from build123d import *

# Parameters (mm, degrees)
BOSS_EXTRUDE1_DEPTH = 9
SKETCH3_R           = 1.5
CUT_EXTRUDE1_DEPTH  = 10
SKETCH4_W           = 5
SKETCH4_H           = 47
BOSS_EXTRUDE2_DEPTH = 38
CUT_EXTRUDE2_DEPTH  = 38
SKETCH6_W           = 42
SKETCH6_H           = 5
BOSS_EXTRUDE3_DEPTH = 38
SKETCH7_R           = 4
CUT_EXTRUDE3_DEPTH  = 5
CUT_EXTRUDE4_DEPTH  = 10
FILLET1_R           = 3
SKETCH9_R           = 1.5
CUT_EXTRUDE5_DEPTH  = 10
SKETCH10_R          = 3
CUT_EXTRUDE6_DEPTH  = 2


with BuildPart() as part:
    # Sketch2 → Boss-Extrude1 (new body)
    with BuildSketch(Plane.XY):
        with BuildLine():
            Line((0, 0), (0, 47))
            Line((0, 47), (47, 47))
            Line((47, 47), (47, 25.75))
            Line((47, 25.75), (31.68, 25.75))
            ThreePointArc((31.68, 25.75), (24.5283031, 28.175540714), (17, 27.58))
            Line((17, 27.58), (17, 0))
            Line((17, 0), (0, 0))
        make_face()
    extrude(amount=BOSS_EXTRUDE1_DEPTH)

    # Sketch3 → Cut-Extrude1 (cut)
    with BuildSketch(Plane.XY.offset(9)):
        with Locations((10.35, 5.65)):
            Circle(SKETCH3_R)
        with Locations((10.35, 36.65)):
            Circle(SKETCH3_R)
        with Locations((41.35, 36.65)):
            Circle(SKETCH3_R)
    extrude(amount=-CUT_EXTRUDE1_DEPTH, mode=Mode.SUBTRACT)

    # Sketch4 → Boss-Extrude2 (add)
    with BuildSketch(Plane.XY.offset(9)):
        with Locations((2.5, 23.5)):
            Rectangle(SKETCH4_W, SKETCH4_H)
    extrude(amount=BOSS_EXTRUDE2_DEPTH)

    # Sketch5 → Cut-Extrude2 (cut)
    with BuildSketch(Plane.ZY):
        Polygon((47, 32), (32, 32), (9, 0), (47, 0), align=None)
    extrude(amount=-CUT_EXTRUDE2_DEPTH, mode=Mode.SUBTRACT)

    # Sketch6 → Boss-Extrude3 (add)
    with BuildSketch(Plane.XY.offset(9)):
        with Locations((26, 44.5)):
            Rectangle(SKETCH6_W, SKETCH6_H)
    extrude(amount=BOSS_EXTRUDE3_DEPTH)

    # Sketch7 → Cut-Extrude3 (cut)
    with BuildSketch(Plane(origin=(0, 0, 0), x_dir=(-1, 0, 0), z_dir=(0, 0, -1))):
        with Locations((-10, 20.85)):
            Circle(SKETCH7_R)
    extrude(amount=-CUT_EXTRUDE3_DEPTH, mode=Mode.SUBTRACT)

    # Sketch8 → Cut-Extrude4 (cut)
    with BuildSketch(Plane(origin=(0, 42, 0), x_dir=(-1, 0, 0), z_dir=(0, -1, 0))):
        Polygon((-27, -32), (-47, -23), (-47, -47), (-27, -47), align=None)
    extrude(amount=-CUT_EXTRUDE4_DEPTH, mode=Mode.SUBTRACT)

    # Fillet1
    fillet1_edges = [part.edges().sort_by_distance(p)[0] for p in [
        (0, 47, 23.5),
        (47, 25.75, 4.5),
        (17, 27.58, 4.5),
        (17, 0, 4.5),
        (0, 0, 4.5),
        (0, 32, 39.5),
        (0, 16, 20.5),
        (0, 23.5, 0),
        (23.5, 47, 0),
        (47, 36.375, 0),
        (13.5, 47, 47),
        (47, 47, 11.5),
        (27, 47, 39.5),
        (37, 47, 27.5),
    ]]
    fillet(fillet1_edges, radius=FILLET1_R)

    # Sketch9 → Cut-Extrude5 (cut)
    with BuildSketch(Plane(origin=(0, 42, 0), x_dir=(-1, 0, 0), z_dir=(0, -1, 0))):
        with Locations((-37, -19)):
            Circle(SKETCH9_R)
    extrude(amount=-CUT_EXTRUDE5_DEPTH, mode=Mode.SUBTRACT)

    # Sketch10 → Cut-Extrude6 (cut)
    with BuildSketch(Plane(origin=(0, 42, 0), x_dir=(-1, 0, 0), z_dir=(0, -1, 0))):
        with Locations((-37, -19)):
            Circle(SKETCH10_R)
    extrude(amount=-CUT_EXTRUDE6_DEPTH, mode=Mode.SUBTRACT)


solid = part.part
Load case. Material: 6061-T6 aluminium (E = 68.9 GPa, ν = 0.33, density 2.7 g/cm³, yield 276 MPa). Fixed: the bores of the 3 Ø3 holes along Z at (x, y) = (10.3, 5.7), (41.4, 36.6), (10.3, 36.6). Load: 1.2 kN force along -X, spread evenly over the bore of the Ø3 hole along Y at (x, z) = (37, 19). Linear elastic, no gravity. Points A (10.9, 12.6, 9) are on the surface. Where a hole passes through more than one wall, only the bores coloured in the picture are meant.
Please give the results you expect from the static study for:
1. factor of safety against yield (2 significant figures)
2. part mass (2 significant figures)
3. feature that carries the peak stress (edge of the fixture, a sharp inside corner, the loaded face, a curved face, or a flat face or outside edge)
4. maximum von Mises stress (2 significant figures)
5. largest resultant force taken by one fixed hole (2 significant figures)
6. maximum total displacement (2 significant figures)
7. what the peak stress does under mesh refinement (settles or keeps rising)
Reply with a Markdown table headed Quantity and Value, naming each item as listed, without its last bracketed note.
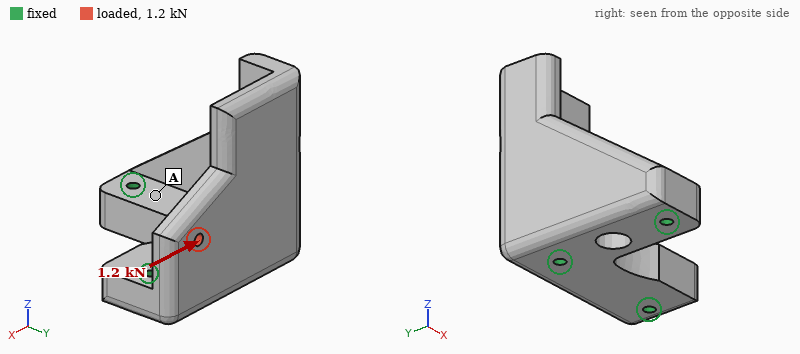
| Quantity | Value |
|---|---|
| factor of safety against yield | 3.7 |
| part mass | 60 g |
| feature that carries the peak stress | the loaded face |
| maximum von Mises stress | 75 MPa |
| largest resultant force taken by one fixed hole | 850 N |
| maximum total displacement | 11 µm |
| what the peak stress does under mesh refinement | settles |
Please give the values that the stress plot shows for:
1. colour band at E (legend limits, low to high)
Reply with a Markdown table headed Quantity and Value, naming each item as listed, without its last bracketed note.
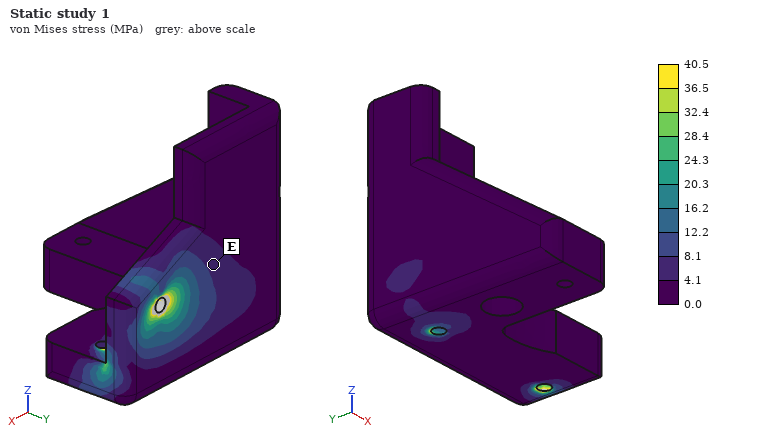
| Quantity | Value |
|---|---|
| colour band at E | 4.1 to 8.1 MPa |
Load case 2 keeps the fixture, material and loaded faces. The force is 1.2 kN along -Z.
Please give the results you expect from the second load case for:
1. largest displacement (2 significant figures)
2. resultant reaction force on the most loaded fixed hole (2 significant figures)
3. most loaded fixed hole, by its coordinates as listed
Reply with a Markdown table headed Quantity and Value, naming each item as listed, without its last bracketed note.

| Quantity | Value |
|---|---|
| largest displacement | 22 µm |
| resultant reaction force on the most loaded fixed hole | 990 N |
| most loaded fixed hole, by its coordinates as listed | (41.4, 36.6) |
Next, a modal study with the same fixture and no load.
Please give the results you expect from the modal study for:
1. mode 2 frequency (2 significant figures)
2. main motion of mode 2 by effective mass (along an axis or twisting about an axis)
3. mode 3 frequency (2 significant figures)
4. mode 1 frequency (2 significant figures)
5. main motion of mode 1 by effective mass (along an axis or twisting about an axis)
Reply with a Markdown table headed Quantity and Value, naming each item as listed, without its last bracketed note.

| Quantity | Value |
|---|---|
| mode 2 frequency | 8300 Hz |
| main motion of mode 2 by effective mass | along X |
| mode 3 frequency | 13 kHz |
| mode 1 frequency | 5800 Hz |
| main motion of mode 1 by effective mass | along Y |
